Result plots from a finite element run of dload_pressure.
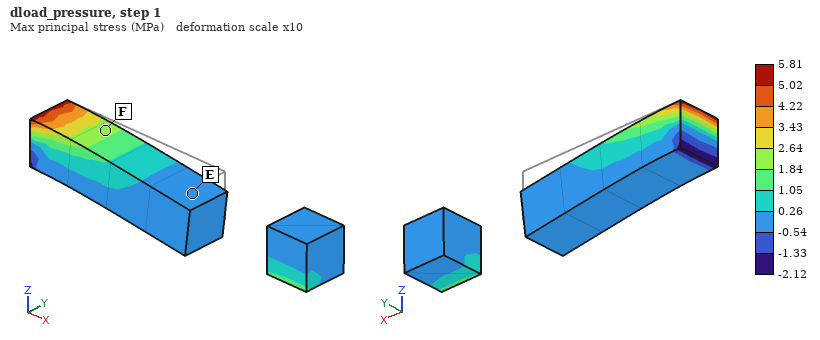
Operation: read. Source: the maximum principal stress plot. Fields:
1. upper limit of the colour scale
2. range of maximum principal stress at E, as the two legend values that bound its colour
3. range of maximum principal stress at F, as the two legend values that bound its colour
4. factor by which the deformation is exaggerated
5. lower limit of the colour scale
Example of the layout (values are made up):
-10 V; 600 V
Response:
5.81 MPa; -0.54 to 0.26 MPa; 1.84 to 2.64 MPa; 10; -2.12 MPa
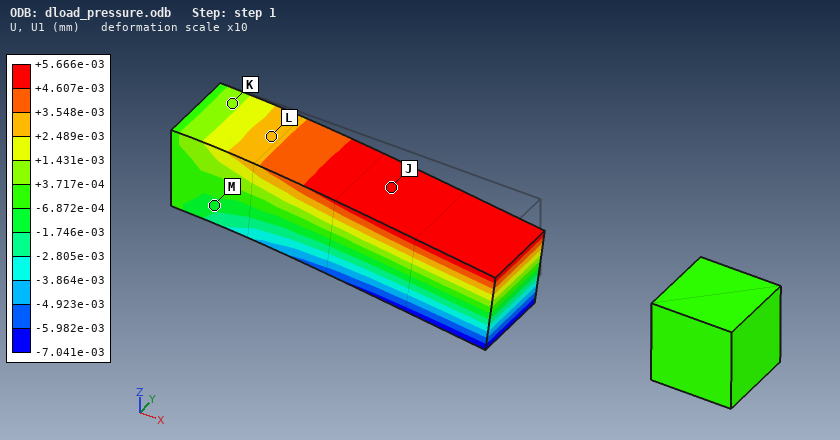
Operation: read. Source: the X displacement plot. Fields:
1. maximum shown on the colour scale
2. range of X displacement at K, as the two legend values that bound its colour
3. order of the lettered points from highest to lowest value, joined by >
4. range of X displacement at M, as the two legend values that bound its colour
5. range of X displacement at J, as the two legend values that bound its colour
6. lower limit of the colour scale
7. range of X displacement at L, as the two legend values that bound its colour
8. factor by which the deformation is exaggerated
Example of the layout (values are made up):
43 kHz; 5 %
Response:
+5.666e-03 mm; +3.717e-04 to +1.431e-03 mm; J > L > K > M; -1.746e-03 to -6.872e-04 mm; +4.607e-03 to +5.666e-03 mm; -7.041e-03 mm; +2.489e-03 to +3.548e-03 mm; 10
